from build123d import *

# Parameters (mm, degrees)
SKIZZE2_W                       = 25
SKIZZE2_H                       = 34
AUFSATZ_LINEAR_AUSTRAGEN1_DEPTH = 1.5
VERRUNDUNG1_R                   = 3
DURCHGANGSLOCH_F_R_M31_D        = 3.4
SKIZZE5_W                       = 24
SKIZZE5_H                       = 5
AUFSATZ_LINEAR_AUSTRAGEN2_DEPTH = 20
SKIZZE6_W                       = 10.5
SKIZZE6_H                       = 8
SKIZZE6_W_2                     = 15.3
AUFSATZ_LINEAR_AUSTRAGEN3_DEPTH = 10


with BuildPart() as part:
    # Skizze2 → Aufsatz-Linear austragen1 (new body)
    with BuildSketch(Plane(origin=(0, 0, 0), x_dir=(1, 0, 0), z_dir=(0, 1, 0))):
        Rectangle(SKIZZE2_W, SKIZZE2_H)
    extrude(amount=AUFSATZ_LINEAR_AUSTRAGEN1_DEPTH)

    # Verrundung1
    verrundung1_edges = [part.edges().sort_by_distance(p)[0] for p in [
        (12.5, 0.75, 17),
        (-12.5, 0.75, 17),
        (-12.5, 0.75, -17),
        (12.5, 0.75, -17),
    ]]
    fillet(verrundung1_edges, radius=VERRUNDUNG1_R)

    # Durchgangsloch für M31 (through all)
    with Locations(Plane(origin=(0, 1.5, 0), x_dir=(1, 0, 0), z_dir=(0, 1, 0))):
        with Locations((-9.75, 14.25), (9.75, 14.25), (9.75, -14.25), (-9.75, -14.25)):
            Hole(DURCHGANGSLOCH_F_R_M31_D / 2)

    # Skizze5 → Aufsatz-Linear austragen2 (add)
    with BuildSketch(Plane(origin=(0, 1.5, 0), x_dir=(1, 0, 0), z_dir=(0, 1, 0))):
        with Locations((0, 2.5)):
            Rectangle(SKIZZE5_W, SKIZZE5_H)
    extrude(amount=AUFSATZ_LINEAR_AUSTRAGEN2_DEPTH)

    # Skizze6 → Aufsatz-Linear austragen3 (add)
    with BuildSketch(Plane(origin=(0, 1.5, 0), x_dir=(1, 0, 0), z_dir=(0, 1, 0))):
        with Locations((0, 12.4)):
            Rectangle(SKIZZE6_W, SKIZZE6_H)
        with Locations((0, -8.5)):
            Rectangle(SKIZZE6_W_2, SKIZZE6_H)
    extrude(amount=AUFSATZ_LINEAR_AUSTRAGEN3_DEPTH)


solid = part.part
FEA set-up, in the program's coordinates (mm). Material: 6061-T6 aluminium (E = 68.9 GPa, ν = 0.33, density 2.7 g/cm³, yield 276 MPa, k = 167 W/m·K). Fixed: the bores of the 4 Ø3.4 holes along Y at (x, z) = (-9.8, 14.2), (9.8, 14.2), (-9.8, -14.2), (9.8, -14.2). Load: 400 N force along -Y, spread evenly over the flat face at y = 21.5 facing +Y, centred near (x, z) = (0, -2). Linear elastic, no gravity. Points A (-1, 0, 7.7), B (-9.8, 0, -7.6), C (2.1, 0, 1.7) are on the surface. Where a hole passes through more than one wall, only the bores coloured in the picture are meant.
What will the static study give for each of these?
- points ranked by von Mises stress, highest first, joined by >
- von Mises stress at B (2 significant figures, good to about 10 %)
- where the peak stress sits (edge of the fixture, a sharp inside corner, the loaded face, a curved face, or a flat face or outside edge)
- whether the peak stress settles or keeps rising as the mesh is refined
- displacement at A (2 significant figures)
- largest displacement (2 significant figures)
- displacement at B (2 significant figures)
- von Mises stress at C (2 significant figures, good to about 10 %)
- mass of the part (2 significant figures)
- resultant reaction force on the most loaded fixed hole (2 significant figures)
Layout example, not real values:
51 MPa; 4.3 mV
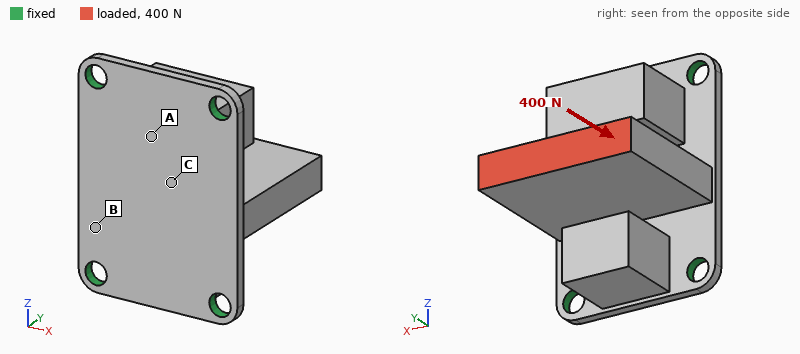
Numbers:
C > B > A; 27 MPa; edge of the fixture; keeps rising; 26 µm; 71 µm; 29 µm; 71 MPa; 15 g; 130 N
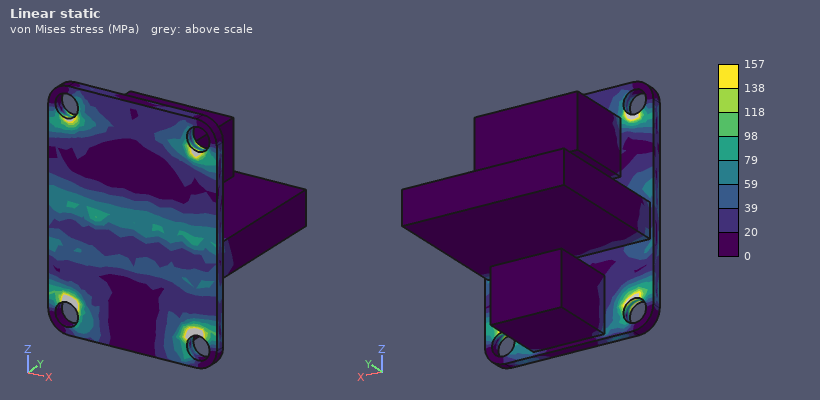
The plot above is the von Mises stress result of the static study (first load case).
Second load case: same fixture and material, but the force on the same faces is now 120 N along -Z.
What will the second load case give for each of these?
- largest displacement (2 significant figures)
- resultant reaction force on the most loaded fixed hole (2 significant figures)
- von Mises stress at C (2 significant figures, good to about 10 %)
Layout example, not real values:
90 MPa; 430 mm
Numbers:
0.12 mm; 74 N; 76 MPa
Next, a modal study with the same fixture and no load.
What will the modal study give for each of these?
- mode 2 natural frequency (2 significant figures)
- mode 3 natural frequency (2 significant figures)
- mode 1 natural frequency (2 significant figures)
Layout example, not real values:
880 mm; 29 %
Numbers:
4900 Hz; 5000 Hz; 3100 Hz
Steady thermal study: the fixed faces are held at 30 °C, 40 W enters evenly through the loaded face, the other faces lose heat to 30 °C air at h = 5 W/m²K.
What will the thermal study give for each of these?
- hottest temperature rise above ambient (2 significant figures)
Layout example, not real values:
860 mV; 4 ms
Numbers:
77 K
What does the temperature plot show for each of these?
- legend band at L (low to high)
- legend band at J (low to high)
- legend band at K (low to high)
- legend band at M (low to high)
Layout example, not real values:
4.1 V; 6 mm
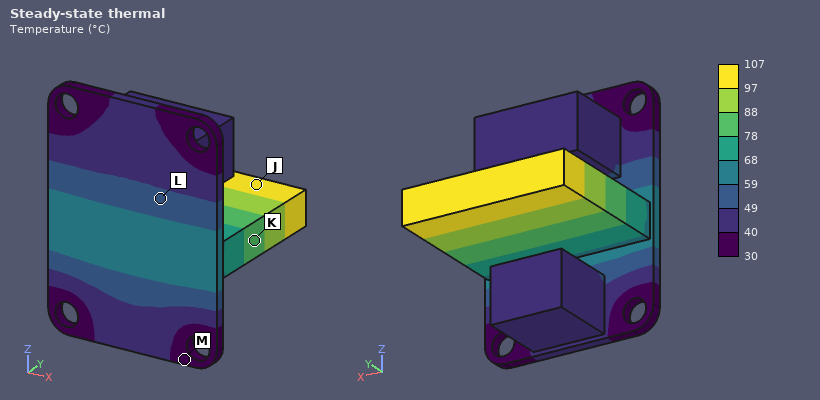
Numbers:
49 to 59 °C; 97 to 107 °C; 78 to 88 °C; 30 to 40 °C
